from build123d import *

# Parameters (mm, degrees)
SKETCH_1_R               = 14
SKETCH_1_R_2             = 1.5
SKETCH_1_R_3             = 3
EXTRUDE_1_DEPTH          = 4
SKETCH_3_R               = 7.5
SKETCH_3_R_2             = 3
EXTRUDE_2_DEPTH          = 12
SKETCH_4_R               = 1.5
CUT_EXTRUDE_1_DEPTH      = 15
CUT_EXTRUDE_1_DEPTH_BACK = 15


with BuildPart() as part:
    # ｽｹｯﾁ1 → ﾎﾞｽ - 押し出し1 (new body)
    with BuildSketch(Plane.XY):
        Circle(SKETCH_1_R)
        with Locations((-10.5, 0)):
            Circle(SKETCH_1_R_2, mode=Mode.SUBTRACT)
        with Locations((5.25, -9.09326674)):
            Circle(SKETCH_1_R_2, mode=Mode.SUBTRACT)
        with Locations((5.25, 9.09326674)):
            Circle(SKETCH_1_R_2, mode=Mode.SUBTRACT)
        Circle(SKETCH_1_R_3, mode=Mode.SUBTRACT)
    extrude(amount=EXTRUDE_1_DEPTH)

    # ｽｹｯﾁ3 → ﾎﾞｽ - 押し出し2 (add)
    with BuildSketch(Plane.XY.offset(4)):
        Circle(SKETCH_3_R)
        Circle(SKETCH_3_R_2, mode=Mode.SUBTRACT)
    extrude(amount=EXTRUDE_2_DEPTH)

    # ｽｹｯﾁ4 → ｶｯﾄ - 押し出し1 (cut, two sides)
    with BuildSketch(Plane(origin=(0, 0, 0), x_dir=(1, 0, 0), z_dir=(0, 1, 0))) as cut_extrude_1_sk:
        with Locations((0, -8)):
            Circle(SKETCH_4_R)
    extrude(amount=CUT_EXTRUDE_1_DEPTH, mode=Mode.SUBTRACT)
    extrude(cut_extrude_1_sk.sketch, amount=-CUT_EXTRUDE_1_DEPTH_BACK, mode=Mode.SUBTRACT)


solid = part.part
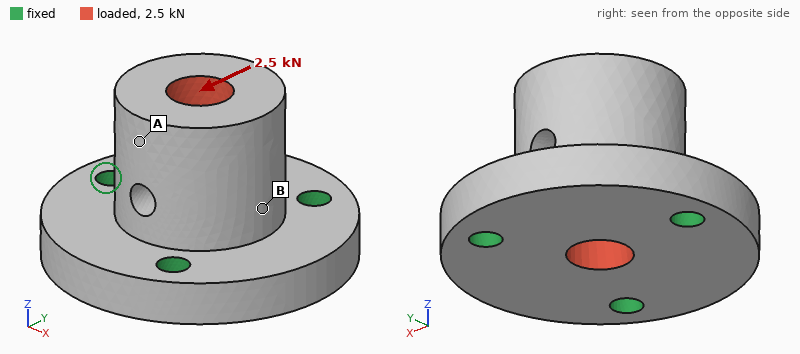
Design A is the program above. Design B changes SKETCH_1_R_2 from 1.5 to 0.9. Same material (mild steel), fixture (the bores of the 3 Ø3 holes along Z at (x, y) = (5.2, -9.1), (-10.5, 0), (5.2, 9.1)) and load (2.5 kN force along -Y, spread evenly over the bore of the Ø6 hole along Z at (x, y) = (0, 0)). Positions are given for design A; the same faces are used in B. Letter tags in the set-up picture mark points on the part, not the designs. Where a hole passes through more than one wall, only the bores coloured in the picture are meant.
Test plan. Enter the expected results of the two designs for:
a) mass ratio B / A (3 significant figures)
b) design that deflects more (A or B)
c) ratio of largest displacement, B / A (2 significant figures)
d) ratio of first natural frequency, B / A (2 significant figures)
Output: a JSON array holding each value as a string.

["1.01", "B", "1.2", "0.90"]
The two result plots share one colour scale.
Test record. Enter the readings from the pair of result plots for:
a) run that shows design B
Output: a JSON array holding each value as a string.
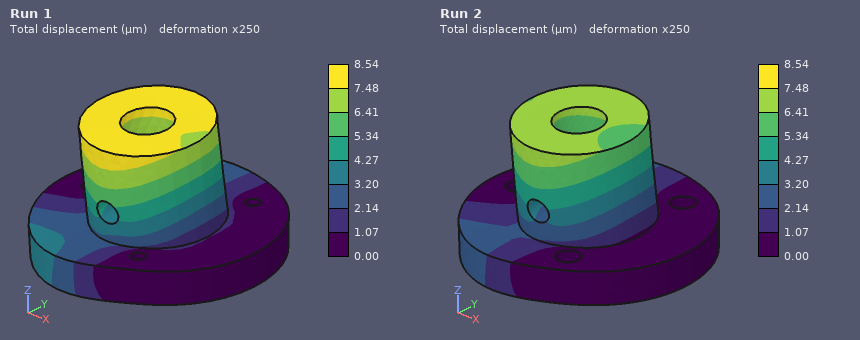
["Run 1"]
